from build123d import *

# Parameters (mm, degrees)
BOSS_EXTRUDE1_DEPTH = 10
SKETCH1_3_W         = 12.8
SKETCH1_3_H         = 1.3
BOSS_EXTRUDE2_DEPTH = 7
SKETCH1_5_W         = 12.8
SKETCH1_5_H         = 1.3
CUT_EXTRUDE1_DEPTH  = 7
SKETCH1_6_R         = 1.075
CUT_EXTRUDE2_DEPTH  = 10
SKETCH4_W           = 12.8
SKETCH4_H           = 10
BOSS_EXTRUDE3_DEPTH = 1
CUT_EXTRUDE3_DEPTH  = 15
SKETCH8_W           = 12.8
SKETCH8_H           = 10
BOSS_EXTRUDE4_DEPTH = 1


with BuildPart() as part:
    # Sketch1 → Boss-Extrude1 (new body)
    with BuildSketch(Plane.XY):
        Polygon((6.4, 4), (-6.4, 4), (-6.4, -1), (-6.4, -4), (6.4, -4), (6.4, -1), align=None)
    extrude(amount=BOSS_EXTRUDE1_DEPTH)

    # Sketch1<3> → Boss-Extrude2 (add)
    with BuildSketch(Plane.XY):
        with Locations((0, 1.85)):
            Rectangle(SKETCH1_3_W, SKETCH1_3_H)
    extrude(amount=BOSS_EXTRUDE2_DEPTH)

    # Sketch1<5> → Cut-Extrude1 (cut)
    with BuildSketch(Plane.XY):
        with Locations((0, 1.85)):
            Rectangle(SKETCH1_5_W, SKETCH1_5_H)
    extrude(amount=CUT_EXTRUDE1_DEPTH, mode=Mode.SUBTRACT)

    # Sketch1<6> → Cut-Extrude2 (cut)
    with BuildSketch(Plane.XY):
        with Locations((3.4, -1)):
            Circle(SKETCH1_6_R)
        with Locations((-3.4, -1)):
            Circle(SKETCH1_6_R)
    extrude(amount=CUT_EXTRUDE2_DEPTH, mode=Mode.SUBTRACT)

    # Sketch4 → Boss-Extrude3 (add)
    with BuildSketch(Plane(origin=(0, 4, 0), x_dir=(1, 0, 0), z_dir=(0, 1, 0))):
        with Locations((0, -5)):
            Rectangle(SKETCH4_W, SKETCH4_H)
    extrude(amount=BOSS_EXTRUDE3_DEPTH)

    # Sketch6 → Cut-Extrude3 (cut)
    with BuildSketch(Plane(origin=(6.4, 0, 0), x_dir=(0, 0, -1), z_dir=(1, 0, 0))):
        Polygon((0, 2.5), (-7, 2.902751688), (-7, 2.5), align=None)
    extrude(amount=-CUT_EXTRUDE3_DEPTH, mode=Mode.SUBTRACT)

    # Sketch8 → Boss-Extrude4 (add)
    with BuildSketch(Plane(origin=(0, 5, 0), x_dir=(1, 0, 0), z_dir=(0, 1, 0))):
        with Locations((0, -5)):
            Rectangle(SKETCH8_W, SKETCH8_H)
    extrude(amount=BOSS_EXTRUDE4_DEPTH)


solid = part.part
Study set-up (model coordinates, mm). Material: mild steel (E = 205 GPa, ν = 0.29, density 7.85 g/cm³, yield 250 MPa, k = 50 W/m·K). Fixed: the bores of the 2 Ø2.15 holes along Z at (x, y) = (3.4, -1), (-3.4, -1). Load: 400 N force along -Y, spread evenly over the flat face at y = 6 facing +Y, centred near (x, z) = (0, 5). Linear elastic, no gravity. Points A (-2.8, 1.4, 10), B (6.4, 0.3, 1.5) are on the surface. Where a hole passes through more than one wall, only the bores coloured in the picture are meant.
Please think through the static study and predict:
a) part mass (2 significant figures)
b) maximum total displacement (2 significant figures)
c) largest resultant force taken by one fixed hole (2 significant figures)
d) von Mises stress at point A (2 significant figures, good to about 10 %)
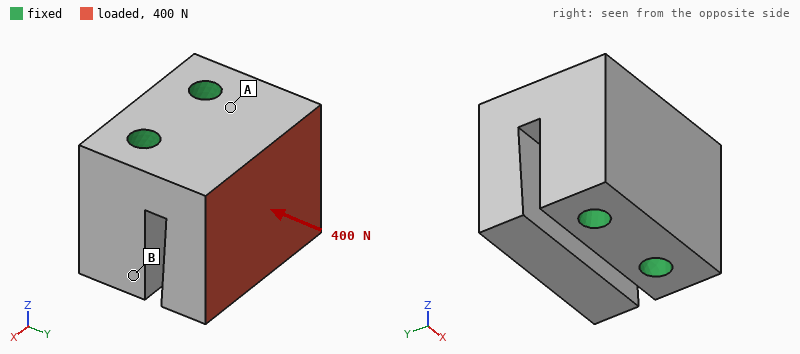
8.4 g
11 µm
200 N
56 MPa
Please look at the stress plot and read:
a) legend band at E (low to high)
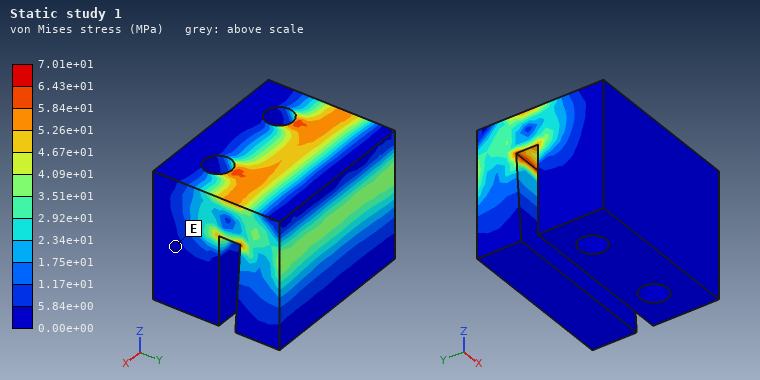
0.00e+00 to 5.84e+00 MPa
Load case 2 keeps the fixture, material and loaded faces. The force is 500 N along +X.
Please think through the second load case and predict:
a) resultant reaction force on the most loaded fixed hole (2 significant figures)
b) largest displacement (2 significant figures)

480 N
4.9 µm
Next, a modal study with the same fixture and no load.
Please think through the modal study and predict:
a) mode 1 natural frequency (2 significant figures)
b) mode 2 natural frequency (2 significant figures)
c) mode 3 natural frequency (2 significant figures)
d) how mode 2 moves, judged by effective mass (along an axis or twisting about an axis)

18 kHz
31 kHz
47 kHz
along X
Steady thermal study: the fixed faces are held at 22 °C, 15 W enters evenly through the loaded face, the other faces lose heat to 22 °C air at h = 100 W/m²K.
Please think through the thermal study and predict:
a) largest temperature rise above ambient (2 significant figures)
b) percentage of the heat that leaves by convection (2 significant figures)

53 K
7.6 %
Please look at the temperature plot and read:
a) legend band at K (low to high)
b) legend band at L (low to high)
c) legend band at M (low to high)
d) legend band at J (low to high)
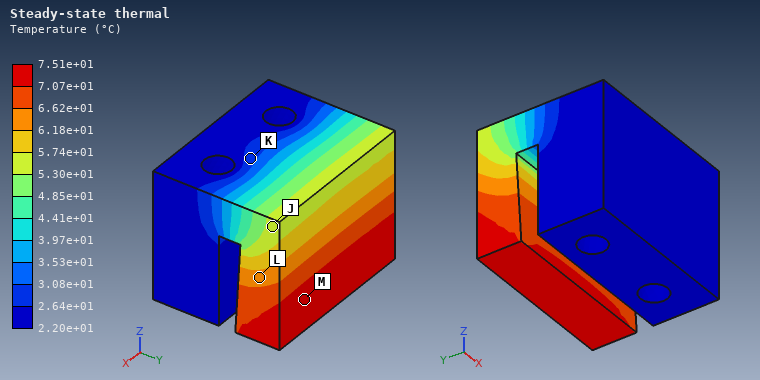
2.64e+01 to 3.08e+01 °C
6.18e+01 to 6.62e+01 °C
7.07e+01 to 7.51e+01 °C
5.30e+01 to 5.74e+01 °C
